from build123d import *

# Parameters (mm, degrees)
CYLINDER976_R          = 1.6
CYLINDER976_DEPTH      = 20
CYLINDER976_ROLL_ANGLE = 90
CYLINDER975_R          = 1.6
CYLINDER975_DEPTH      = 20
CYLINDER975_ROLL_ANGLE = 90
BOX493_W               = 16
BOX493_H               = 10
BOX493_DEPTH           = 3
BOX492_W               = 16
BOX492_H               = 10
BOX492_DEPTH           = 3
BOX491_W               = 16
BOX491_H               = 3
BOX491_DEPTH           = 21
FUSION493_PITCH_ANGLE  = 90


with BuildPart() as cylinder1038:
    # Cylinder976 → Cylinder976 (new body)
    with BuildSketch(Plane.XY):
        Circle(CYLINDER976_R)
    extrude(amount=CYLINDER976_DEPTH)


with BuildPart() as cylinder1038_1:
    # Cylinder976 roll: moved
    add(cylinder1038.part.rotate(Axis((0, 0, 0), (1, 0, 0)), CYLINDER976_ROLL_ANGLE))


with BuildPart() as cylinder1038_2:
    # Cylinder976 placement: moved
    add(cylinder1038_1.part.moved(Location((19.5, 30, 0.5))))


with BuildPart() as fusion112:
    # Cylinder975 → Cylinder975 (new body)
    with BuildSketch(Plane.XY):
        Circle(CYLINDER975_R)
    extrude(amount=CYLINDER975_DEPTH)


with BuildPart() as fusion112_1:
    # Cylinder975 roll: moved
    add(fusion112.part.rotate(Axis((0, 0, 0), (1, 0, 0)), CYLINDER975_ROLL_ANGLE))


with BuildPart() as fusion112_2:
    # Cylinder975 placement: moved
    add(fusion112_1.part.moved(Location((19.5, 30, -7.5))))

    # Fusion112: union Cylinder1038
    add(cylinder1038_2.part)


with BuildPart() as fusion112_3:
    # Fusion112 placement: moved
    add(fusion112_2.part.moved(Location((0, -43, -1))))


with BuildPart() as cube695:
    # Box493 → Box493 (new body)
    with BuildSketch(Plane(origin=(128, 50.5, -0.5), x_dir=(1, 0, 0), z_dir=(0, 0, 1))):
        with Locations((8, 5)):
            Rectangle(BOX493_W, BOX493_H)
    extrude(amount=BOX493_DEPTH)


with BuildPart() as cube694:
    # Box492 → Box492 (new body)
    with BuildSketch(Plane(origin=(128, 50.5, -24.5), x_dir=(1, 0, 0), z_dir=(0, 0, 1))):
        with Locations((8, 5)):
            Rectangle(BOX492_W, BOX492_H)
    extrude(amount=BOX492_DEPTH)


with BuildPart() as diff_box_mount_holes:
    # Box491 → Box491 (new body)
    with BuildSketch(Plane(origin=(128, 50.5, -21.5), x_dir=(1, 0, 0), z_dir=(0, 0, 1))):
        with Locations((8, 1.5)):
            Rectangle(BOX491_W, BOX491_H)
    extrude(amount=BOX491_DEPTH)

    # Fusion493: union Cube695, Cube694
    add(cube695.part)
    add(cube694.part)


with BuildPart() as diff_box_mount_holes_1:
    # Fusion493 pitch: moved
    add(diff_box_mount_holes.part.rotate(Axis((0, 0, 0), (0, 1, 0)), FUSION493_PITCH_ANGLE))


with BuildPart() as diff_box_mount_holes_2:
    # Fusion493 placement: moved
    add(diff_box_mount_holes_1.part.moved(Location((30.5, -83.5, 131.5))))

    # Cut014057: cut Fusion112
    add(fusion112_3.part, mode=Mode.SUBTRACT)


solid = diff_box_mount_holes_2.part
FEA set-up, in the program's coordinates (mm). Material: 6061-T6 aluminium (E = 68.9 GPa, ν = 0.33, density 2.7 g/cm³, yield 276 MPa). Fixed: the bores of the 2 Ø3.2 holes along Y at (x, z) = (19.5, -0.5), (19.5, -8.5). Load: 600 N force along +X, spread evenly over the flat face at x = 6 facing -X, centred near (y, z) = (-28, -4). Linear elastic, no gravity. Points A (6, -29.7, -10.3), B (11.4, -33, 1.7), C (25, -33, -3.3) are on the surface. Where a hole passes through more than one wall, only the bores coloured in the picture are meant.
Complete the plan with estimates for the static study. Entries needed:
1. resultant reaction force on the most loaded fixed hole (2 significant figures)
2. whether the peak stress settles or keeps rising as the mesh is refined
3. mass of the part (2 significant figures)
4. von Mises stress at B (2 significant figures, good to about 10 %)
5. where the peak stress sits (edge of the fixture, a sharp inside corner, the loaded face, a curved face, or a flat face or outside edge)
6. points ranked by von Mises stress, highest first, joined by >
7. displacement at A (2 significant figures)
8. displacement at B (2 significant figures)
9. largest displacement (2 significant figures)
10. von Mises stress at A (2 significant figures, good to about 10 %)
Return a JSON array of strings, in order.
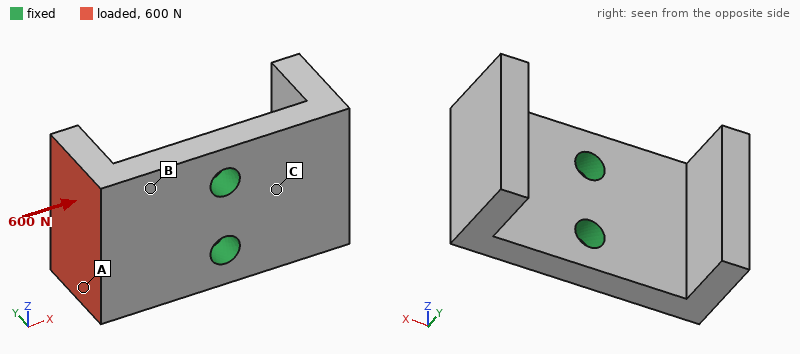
["300 N", "keeps rising", "5.2 g", "75 MPa", "edge of the fixture", "B > A > C", "0.067 mm", "0.022 mm", "0.11 mm", "48 MPa"]
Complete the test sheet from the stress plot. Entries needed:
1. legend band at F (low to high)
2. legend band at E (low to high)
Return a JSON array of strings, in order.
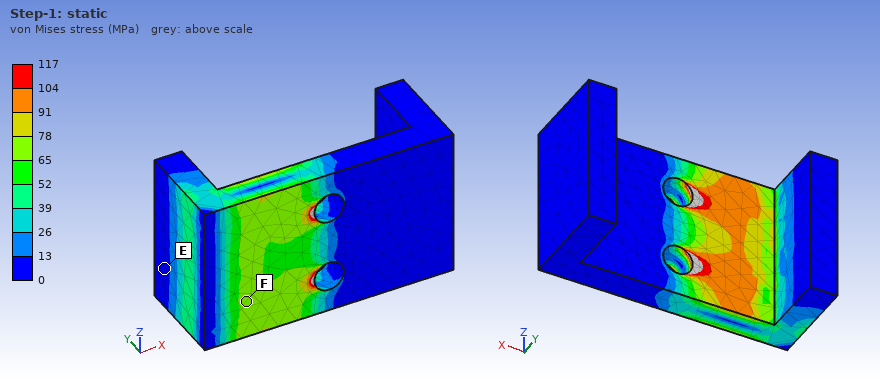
["65 to 78 MPa", "0 to 13 MPa"]
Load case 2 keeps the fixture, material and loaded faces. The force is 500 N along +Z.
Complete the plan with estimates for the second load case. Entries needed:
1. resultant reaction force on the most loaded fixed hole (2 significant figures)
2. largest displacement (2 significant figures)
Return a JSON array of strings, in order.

["700 N", "44 µm"]
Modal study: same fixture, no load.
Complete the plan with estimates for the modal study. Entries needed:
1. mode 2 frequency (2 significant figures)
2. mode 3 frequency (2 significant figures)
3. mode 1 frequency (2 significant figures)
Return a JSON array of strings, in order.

["8300 Hz", "14 kHz", "8100 Hz"]
